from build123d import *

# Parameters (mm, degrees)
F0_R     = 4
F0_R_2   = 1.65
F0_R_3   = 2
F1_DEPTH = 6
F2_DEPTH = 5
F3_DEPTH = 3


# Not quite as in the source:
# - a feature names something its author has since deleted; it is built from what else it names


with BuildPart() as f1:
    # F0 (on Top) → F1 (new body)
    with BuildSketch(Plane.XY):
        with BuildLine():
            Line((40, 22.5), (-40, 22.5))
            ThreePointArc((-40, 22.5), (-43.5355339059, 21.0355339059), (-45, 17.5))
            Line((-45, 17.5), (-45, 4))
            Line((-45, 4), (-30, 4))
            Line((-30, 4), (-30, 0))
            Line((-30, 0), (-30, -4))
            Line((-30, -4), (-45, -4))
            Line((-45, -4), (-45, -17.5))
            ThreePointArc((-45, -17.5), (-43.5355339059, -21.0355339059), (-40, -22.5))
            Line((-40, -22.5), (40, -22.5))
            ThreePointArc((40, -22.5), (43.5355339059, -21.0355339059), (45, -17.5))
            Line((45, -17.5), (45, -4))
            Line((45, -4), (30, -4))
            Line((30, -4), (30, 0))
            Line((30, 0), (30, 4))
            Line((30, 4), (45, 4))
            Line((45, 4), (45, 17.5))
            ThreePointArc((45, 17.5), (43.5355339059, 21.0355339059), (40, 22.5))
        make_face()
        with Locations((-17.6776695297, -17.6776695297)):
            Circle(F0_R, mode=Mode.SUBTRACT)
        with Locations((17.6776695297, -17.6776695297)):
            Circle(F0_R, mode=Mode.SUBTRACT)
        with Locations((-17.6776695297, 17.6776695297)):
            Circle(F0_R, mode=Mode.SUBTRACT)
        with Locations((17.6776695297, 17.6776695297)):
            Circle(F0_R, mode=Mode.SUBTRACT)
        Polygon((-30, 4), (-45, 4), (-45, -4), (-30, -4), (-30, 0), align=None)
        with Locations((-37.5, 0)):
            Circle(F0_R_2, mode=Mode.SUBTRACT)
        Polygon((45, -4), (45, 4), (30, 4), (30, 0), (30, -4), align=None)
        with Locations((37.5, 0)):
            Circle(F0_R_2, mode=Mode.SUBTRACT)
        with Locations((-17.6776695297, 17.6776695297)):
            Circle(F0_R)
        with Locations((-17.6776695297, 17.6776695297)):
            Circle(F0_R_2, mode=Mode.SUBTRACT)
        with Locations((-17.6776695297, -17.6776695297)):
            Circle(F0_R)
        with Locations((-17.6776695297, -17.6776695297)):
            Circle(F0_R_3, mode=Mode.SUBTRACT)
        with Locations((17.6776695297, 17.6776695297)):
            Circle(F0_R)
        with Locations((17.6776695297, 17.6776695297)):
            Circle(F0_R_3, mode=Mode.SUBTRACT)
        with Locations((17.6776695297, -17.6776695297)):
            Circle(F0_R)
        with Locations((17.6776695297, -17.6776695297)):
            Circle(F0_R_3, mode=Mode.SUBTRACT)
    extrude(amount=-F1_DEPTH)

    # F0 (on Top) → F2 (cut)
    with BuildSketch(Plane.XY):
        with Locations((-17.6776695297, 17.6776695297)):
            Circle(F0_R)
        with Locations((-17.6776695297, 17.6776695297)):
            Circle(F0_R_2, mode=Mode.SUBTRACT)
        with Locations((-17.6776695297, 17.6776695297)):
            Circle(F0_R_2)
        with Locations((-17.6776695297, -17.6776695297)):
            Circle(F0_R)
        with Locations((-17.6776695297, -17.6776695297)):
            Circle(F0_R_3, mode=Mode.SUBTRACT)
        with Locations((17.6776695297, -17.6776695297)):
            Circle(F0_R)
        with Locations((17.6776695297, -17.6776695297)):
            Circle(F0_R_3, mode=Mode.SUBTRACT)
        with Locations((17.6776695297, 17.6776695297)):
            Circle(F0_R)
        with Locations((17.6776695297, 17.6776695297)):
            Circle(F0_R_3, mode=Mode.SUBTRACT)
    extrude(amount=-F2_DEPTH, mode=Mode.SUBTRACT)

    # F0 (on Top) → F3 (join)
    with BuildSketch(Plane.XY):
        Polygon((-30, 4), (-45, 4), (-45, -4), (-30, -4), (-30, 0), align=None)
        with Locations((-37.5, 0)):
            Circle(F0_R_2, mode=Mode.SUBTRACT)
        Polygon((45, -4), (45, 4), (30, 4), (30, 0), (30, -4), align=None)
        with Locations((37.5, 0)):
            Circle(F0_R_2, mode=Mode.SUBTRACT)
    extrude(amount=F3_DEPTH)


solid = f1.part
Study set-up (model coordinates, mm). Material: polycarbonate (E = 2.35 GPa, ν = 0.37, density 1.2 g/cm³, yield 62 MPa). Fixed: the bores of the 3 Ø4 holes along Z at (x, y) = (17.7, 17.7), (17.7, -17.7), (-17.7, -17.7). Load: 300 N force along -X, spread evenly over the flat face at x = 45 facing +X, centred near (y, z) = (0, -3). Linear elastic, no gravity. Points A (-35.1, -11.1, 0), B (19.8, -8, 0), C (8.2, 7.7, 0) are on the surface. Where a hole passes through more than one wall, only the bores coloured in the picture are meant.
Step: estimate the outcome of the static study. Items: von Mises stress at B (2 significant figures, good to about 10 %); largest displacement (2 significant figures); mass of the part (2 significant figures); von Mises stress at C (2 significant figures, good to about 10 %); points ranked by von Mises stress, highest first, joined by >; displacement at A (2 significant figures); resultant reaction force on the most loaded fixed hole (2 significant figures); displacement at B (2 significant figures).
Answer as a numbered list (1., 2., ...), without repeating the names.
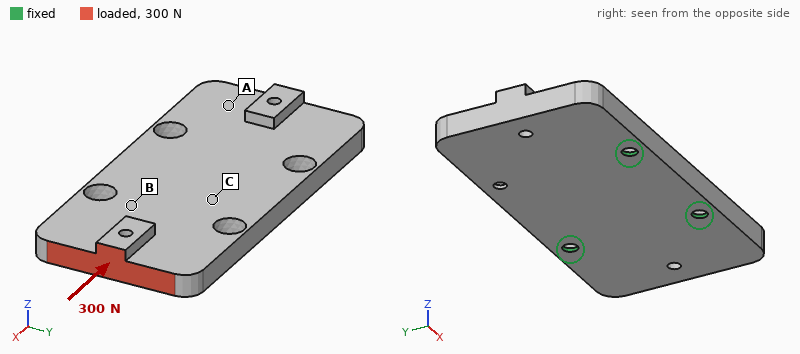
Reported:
1. 3.1 MPa
2. 0.21 mm
3. 28 g
4. 1.8 MPa
5. B > C > A
6. 0.046 mm
7. 110 N
8. 0.049 mm
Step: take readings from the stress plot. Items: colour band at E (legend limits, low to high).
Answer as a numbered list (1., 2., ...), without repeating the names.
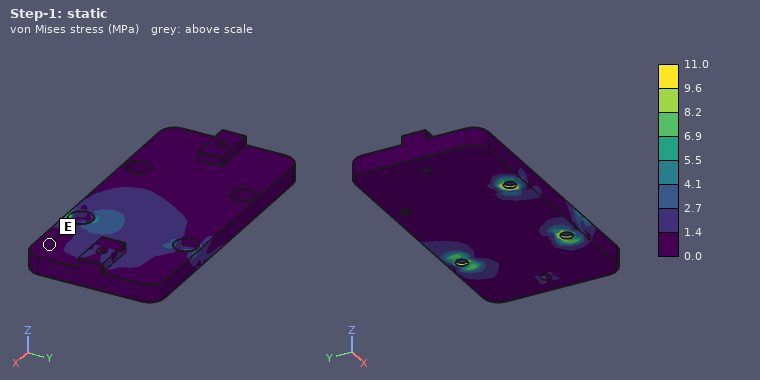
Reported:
1. 0.0 to 1.4 MPa
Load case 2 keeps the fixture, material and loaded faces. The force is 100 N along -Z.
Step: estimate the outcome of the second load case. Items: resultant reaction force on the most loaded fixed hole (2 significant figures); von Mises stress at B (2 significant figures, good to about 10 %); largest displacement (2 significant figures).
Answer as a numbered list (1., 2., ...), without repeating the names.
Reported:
1. 190 N
2. 11 MPa
3. 1.0 mm
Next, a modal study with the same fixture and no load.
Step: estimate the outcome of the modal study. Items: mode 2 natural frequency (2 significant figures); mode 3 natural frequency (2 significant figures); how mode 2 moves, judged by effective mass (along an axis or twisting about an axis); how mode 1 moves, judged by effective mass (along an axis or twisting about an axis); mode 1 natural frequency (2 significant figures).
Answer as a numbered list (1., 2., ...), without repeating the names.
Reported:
1. 960 Hz
2. 1500 Hz
3. along Z
4. along Z
5. 520 Hz
